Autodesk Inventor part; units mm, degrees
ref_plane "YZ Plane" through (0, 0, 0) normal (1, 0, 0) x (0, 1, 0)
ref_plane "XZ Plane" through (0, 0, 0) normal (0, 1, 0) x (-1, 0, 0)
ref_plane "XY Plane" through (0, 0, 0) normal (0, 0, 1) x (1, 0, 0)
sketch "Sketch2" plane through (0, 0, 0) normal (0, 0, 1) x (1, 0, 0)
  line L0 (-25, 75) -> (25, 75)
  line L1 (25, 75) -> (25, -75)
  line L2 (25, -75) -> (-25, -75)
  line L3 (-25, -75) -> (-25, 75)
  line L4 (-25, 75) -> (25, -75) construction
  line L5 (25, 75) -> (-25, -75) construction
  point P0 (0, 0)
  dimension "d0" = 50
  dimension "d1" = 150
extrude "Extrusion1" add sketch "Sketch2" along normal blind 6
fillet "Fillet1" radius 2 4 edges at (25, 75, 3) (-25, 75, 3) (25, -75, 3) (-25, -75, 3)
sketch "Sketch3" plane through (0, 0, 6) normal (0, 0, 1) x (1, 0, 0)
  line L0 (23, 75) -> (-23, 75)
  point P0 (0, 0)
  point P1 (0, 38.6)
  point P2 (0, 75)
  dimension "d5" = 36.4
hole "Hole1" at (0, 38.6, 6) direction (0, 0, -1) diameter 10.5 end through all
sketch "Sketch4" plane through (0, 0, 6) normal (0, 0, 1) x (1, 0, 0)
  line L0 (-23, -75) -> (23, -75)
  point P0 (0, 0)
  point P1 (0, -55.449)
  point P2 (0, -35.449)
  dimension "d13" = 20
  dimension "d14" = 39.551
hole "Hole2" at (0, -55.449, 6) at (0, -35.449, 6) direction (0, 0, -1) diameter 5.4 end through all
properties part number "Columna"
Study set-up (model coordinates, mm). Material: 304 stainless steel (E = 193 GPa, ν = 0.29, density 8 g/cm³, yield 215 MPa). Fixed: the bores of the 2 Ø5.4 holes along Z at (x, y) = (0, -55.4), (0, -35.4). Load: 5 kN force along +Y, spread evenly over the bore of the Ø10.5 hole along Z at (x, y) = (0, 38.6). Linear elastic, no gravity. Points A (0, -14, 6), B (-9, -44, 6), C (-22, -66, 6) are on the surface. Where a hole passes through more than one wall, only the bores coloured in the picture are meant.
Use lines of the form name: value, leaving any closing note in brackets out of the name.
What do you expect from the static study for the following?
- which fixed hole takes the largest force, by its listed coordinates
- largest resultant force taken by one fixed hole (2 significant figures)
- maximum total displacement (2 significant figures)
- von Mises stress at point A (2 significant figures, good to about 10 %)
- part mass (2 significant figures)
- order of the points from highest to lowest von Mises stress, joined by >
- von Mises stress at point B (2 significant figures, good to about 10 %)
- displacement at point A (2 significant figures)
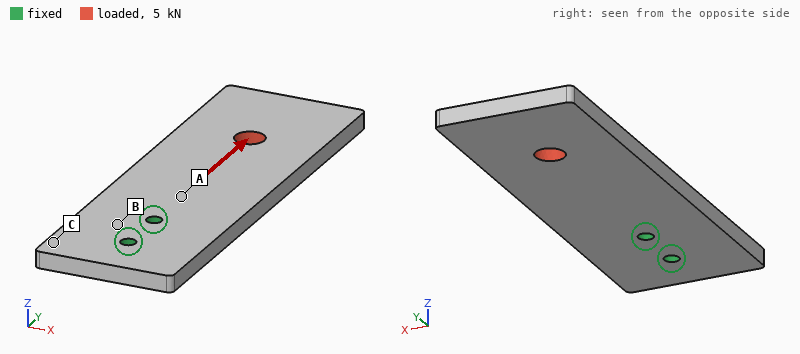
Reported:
which fixed hole takes the largest force, by its listed coordinates: (0, -35.4)
largest resultant force taken by one fixed hole: 3.5 kN
maximum total displacement: 9.4 µm
von Mises stress at point A: 21 MPa
part mass: 350 g
order of the points from highest to lowest von Mises stress, joined by >: A > B > C
von Mises stress at point B: 12 MPa
displacement at point A: 2.9 µm
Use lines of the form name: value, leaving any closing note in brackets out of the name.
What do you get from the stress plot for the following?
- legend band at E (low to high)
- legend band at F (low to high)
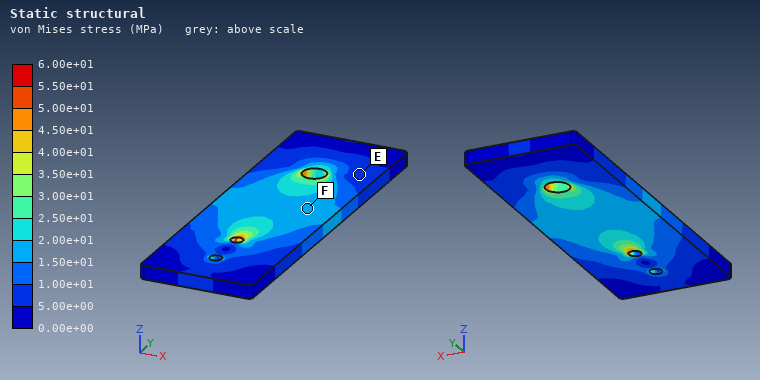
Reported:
legend band at E: 5.00e+00 to 1.00e+01 MPa
legend band at F: 1.50e+01 to 2.00e+01 MPa
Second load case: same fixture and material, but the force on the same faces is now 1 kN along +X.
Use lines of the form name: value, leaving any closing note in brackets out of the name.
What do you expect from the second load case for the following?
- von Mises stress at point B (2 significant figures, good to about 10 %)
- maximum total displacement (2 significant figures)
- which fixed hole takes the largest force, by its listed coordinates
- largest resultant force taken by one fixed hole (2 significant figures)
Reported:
von Mises stress at point B: 25 MPa
maximum total displacement: 53 µm
which fixed hole takes the largest force, by its listed coordinates: (0, -35.4)
largest resultant force taken by one fixed hole: 3.9 kN
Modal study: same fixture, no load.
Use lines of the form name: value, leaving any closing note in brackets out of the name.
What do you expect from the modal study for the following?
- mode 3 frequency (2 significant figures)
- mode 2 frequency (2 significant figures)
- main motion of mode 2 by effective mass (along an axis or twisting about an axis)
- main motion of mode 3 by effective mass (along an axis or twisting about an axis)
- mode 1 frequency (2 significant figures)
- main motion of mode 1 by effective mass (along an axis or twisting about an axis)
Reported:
mode 3 frequency: 1900 Hz
mode 2 frequency: 1500 Hz
main motion of mode 2 by effective mass: twisting about Y
main motion of mode 3 by effective mass: along X
mode 1 frequency: 380 Hz
main motion of mode 1 by effective mass: along Z
